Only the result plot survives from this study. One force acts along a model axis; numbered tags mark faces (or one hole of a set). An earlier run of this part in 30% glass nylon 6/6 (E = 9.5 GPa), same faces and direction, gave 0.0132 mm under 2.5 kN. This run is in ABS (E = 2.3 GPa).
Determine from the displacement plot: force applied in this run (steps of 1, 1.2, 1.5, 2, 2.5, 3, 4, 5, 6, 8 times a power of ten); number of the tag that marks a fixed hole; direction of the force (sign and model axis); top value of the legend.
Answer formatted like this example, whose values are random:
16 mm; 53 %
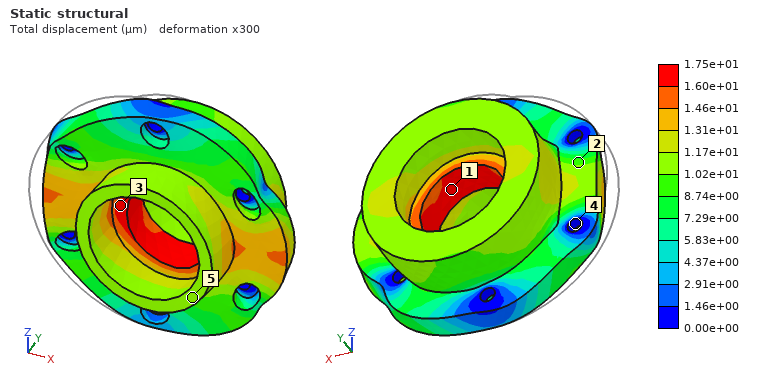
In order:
800 N; 4; +X; 1.75e+01 µm
